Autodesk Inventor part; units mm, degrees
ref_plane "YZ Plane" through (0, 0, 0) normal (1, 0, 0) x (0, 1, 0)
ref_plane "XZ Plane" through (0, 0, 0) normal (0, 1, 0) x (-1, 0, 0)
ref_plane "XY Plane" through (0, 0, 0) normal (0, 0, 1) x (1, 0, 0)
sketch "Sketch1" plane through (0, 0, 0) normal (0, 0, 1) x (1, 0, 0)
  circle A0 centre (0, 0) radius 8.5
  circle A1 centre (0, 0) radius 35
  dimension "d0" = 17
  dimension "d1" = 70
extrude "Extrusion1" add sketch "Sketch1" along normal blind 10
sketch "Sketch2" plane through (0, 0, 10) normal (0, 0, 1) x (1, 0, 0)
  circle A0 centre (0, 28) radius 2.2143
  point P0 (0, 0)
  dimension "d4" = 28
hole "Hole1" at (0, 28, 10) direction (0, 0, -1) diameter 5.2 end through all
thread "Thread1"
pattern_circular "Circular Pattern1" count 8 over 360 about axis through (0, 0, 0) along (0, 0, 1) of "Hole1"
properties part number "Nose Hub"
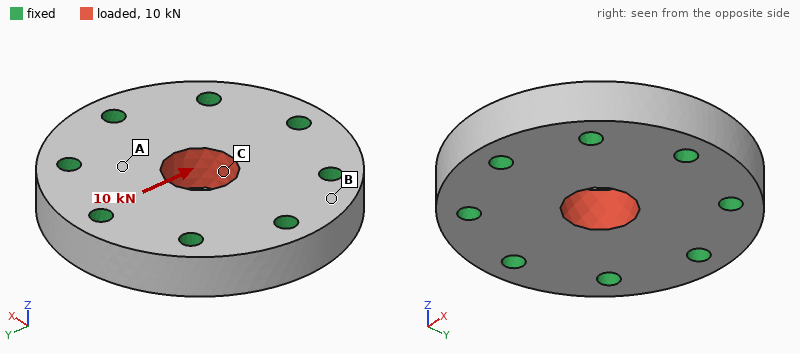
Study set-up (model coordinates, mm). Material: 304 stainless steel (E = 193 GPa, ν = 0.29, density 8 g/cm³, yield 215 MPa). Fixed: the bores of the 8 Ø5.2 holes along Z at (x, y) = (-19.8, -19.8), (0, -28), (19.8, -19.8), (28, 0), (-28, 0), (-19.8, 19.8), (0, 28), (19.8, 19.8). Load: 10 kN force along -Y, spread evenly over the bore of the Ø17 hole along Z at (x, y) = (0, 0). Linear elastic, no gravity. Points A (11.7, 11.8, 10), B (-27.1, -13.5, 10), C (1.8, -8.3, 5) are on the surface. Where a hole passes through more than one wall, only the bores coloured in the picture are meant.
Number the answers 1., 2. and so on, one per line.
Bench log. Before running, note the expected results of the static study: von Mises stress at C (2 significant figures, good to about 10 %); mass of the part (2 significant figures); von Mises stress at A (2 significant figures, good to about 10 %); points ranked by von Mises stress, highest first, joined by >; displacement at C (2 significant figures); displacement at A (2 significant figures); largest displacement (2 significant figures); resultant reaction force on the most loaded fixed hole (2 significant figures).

1. 17 MPa
2. 280 g
3. 13 MPa
4. C > A > B
5. 1.6 µm
6. 0.71 µm
7. 1.7 µm
8. 2.1 kN
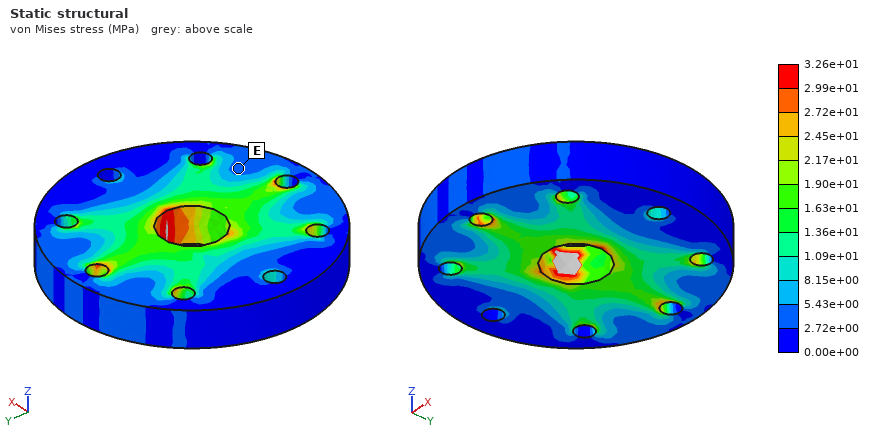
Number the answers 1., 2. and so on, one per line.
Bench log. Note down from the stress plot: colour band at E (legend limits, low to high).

1. 2.72e+00 to 5.43e+00 MPa
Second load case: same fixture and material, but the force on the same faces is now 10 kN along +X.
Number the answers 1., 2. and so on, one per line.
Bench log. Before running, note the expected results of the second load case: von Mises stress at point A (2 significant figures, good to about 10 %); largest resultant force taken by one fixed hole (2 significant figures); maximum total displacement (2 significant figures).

1. 13 MPa
2. 2.1 kN
3. 1.6 µm
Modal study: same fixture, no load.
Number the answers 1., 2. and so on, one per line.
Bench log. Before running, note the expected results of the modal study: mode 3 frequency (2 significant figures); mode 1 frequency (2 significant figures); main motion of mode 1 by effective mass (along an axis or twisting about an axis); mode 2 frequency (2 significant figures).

1. 37 kHz
2. 25 kHz
3. along Z
4. 37 kHz
